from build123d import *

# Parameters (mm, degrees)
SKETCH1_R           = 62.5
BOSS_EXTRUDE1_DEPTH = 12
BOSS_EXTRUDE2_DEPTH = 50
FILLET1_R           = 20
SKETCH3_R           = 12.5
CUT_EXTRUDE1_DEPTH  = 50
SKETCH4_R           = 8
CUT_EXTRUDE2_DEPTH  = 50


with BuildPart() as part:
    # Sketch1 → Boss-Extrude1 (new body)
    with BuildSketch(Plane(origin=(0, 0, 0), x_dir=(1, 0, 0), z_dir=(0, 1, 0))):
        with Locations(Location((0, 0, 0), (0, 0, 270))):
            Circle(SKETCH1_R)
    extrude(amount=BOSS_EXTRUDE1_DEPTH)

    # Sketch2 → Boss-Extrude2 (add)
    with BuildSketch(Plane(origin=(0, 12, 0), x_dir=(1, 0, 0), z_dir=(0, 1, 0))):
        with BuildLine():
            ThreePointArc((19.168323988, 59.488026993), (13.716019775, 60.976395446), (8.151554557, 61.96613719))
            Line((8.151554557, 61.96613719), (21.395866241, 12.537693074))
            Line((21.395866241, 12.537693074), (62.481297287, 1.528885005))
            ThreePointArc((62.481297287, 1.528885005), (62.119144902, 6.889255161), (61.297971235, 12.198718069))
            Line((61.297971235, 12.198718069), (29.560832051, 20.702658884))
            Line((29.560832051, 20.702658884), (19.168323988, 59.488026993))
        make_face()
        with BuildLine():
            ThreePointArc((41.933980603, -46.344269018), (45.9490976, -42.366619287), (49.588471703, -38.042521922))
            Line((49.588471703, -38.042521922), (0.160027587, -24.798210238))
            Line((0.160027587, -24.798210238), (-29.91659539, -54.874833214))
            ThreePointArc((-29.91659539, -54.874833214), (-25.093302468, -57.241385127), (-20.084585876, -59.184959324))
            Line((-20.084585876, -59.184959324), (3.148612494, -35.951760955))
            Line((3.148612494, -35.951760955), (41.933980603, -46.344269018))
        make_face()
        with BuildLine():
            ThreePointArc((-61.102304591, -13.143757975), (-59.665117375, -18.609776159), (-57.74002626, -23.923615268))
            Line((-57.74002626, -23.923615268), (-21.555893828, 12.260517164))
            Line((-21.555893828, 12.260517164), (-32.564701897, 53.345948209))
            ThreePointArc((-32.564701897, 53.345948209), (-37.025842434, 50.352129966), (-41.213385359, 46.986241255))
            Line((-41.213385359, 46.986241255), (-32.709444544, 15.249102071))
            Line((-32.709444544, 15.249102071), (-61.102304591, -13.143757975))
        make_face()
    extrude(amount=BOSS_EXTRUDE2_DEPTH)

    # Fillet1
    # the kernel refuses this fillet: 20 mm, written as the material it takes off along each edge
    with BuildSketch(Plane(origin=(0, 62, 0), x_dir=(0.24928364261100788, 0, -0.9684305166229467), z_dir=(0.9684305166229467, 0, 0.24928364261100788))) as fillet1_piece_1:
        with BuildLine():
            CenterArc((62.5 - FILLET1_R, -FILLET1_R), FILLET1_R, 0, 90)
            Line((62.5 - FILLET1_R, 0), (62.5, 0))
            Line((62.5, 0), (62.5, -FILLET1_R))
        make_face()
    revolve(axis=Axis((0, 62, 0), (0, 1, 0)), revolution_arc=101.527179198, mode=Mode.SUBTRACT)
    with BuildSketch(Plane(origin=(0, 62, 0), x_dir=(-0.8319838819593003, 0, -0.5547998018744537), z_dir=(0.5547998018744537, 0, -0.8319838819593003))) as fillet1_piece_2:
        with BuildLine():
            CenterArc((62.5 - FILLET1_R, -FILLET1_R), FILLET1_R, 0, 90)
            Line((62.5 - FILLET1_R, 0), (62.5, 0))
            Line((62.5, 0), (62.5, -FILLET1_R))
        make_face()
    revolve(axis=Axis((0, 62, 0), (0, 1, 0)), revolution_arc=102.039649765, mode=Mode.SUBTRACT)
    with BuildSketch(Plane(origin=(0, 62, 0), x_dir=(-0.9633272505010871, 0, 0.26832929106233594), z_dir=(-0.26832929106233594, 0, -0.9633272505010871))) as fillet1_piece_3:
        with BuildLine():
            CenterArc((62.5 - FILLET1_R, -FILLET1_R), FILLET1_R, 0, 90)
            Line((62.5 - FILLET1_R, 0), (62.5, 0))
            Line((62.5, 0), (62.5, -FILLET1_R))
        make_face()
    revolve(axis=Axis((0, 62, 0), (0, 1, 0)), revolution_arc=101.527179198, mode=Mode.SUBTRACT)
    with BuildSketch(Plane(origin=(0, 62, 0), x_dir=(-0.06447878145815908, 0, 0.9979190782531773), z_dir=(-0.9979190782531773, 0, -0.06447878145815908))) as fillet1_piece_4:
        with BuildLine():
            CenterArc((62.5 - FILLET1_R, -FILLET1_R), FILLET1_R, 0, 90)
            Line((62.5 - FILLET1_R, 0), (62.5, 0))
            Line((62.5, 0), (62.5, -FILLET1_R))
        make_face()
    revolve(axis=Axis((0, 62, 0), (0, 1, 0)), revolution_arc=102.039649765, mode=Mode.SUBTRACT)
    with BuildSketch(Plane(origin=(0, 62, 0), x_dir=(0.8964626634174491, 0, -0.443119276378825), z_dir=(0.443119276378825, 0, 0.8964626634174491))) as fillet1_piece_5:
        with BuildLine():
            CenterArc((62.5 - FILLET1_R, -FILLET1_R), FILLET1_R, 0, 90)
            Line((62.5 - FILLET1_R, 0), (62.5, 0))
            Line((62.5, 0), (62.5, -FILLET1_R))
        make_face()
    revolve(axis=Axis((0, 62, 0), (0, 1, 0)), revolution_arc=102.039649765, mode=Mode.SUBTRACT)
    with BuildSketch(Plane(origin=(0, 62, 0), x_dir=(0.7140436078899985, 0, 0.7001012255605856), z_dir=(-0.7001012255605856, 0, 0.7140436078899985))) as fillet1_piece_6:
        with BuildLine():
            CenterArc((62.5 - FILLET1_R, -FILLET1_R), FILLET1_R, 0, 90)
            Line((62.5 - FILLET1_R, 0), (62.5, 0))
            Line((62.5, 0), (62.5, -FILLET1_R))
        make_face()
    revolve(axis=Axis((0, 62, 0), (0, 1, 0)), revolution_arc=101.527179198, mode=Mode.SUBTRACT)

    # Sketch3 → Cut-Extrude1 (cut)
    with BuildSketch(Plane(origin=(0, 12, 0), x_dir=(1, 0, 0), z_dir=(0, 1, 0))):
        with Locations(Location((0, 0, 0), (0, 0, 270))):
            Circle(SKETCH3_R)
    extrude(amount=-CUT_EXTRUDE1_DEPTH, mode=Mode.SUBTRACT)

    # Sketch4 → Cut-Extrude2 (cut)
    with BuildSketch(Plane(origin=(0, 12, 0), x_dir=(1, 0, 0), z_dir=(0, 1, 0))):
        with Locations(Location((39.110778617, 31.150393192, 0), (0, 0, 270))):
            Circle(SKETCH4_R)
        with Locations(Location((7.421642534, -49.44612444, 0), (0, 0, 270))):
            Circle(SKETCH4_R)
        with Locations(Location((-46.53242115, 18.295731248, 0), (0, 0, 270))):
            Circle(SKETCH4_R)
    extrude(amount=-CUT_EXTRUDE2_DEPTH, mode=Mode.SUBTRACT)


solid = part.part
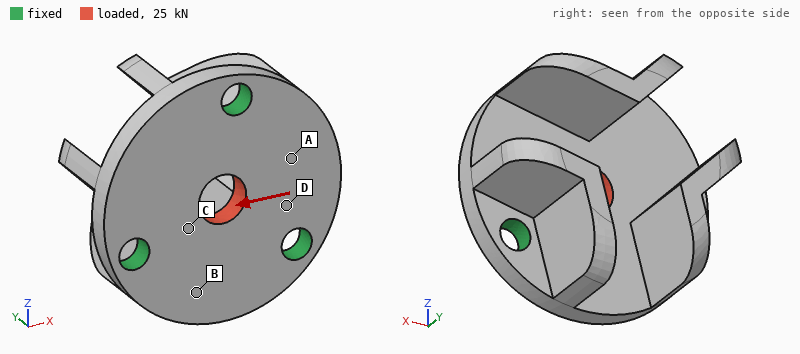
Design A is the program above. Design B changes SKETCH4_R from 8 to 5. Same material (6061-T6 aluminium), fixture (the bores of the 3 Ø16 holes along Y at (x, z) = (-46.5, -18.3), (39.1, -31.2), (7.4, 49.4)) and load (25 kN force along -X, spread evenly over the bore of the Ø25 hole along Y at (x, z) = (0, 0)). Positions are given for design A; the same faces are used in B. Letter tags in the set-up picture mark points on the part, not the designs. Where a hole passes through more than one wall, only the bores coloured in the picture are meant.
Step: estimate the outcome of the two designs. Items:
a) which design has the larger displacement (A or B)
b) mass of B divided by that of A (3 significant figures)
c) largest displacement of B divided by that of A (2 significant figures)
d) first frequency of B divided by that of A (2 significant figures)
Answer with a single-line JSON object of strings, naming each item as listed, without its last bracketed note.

{"which design has the larger displacement": "B", "mass of B divided by that of A": "1.02", "largest displacement of B divided by that of A": "1.1", "first frequency of B divided by that of A": "0.90"}
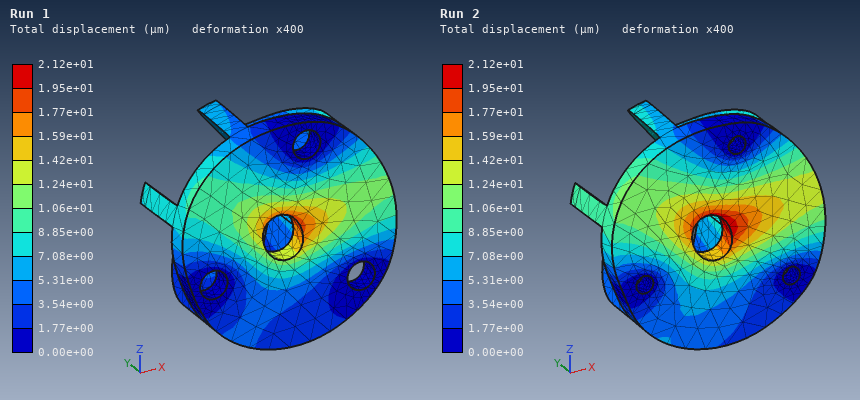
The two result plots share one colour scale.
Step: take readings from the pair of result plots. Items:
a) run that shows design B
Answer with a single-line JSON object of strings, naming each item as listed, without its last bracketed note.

{"run that shows design B": "Run 2"}
